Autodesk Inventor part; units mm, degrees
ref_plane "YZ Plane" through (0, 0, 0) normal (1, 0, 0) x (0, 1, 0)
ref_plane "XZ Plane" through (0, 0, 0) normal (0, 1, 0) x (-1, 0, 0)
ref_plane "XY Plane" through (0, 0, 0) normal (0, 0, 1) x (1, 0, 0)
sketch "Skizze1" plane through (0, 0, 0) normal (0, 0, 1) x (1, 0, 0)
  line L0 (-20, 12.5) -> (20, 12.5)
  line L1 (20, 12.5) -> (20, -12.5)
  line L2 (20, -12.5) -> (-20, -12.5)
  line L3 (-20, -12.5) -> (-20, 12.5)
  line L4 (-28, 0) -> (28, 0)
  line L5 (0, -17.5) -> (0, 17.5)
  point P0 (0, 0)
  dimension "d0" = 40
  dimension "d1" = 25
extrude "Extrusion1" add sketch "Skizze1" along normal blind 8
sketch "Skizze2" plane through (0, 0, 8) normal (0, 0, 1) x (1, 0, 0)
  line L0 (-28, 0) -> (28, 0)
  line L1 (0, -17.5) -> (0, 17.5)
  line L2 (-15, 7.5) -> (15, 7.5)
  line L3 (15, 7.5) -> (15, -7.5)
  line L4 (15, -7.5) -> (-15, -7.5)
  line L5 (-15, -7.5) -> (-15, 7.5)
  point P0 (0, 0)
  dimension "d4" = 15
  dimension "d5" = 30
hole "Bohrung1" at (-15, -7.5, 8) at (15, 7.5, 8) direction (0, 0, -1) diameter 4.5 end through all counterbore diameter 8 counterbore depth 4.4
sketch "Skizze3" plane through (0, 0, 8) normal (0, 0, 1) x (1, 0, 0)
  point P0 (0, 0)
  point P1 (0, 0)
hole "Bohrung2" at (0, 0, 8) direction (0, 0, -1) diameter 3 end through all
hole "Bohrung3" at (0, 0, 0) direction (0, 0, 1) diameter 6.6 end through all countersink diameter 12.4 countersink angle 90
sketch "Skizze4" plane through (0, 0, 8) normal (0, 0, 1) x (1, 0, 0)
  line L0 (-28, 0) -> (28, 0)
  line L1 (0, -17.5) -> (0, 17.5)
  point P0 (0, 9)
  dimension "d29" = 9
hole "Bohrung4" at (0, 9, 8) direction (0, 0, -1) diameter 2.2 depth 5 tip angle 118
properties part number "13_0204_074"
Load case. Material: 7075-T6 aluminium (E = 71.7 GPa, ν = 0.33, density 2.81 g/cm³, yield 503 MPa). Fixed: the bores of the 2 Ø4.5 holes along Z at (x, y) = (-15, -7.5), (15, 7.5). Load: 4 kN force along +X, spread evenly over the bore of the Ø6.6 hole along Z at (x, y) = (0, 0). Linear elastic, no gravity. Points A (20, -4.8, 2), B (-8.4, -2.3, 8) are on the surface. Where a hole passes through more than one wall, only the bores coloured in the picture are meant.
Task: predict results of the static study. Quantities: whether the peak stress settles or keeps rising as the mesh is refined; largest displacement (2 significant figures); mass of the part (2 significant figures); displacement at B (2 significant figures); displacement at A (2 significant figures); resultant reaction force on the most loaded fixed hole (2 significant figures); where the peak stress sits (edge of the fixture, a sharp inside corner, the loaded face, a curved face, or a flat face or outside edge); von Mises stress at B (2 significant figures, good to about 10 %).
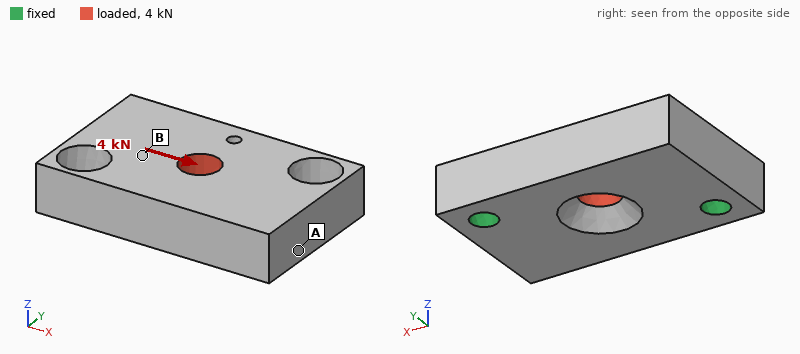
keeps rising
28 µm
20 g
12 µm
17 µm
2.0 kN
edge of the fixture
33 MPa
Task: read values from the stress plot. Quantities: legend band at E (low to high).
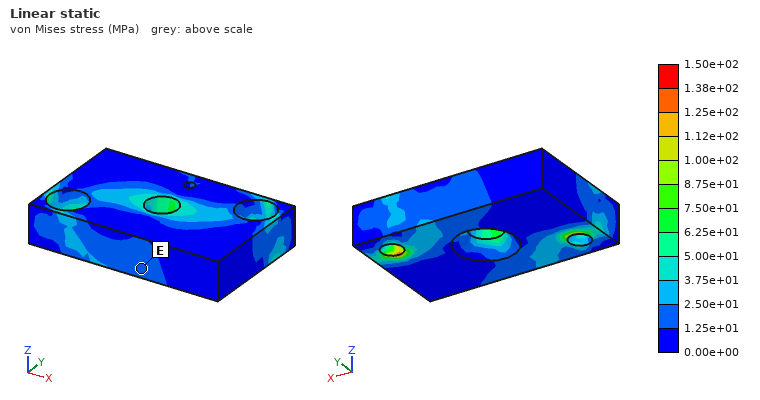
1.25e+01 to 2.50e+01 MPa
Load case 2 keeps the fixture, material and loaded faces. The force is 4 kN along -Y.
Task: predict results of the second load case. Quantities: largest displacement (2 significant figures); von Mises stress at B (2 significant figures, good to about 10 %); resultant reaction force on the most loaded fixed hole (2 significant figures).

52 µm
35 MPa
2.0 kN
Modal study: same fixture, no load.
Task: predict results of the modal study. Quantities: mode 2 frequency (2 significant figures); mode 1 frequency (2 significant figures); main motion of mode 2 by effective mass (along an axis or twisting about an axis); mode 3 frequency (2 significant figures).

15 kHz
8900 Hz
along Z
25 kHz
